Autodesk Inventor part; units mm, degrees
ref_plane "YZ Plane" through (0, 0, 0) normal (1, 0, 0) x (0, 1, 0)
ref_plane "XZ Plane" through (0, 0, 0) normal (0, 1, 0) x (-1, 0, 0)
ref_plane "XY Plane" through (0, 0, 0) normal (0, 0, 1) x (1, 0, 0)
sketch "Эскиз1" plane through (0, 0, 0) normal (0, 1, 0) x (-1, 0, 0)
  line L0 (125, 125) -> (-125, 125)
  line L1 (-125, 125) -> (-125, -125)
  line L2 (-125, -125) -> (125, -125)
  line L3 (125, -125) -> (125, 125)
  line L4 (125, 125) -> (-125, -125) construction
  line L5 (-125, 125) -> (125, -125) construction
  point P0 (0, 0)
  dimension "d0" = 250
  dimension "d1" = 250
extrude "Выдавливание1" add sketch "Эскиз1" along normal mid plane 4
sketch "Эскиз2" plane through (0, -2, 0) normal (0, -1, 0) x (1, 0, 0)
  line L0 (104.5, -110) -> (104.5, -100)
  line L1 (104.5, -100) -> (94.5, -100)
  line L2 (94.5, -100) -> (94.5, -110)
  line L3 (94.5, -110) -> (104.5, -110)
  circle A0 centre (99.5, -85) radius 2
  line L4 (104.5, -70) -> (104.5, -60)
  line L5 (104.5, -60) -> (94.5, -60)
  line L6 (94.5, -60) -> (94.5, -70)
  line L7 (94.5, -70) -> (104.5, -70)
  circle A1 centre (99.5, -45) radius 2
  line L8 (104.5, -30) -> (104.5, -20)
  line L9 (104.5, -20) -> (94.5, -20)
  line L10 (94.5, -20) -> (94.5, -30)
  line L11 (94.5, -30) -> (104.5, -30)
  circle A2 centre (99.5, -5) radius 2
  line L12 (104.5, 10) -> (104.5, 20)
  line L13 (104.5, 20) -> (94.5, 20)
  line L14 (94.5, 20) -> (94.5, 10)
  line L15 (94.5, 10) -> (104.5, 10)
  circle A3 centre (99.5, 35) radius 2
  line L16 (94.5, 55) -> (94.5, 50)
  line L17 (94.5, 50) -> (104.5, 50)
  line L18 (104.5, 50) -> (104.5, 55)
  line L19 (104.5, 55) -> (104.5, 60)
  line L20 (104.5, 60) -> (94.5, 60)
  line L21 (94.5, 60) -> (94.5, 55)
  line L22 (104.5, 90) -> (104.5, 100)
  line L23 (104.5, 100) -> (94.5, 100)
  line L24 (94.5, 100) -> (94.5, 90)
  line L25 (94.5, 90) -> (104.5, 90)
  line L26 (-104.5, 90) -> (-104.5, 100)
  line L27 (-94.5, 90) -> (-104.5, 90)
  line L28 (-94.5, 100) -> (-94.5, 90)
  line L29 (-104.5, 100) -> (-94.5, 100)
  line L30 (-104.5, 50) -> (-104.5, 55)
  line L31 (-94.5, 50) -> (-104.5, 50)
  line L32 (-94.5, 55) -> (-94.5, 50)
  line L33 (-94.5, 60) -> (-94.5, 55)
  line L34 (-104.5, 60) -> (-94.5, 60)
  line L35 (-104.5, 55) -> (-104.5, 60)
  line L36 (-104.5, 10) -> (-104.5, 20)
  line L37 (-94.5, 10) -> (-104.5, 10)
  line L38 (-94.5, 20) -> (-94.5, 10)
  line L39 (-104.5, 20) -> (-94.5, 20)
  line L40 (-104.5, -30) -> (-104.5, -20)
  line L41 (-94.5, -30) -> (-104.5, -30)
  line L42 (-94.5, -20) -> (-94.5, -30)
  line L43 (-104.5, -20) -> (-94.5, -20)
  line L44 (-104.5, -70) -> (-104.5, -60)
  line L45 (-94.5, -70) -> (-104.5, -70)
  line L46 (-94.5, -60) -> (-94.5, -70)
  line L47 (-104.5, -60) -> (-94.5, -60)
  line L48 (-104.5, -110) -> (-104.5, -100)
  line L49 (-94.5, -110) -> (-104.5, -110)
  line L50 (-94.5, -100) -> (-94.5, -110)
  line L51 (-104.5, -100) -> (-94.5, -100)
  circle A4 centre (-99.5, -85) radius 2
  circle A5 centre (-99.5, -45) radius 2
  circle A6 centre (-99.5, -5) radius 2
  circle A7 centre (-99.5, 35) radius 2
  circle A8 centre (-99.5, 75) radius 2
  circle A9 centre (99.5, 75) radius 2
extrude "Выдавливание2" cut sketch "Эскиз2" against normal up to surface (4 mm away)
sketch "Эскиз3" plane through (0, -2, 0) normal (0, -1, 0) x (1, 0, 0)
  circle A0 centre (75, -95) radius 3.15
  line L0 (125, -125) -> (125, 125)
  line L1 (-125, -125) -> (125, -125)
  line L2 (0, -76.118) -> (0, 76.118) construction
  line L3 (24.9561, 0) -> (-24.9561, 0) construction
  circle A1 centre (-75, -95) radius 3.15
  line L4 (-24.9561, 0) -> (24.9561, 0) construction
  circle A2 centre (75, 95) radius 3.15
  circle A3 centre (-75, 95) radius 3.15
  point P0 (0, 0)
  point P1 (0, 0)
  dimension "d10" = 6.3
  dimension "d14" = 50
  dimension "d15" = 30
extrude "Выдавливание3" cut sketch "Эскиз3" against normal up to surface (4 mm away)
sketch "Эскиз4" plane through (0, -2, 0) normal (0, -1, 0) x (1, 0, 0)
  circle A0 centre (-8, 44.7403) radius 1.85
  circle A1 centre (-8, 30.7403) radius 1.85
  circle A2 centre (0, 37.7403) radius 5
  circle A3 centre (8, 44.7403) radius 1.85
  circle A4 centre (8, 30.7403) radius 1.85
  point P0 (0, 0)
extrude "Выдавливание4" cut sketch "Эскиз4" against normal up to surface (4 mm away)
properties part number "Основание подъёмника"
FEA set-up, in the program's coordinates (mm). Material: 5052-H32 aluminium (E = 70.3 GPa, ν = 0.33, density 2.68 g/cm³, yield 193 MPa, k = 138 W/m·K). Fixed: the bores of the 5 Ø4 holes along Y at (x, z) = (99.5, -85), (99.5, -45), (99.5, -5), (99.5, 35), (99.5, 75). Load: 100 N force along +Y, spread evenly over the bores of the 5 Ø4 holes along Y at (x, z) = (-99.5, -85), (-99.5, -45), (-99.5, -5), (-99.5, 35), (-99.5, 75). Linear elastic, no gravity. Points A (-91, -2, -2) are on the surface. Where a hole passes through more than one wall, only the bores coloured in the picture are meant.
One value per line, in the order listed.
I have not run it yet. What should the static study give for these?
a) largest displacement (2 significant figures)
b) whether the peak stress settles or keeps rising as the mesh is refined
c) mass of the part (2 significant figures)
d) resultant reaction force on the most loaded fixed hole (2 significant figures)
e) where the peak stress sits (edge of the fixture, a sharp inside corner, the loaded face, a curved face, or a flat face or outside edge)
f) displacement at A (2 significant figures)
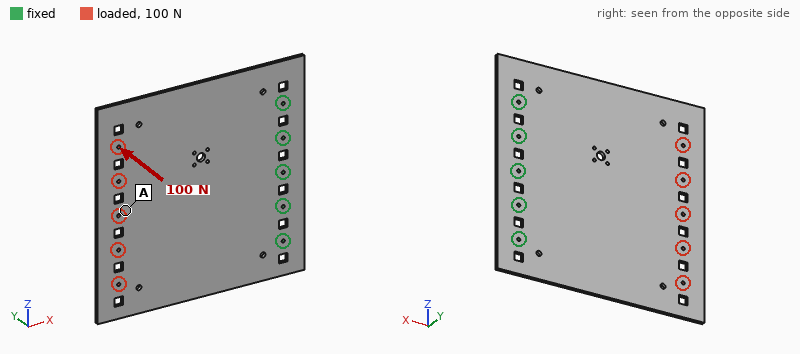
3.6 mm
keeps rising
650 g
46 N
edge of the fixture
2.8 mm
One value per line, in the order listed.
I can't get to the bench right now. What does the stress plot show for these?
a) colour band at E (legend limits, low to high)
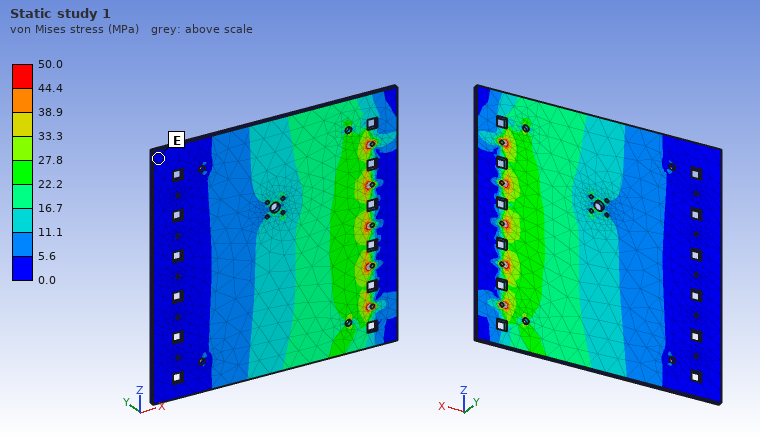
0.0 to 5.6 MPa
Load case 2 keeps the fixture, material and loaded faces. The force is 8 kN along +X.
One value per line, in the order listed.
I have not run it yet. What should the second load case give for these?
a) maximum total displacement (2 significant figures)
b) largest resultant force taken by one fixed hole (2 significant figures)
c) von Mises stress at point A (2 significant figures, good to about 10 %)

34 µm
1.9 kN
17 MPa
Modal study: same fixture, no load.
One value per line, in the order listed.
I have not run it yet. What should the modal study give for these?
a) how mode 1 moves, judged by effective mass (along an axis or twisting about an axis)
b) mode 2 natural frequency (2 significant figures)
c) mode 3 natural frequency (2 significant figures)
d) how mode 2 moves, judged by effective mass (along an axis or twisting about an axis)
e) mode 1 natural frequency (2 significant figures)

along Y
140 Hz
370 Hz
twisting about X
65 Hz
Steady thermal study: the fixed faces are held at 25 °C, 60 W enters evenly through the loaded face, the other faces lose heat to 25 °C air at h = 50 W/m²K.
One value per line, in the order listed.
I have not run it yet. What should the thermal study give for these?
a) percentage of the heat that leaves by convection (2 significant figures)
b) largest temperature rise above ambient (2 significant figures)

92 %
32 K
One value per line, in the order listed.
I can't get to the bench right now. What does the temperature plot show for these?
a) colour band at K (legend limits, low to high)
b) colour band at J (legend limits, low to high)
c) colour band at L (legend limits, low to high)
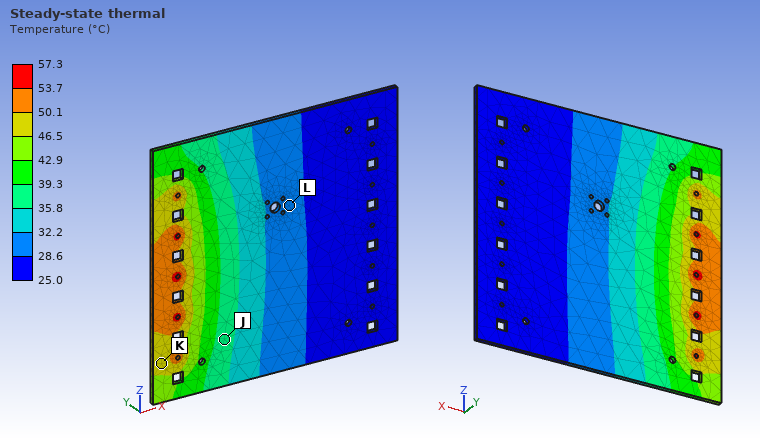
46.5 to 50.1 °C
35.8 to 39.3 °C
28.6 to 32.2 °C
